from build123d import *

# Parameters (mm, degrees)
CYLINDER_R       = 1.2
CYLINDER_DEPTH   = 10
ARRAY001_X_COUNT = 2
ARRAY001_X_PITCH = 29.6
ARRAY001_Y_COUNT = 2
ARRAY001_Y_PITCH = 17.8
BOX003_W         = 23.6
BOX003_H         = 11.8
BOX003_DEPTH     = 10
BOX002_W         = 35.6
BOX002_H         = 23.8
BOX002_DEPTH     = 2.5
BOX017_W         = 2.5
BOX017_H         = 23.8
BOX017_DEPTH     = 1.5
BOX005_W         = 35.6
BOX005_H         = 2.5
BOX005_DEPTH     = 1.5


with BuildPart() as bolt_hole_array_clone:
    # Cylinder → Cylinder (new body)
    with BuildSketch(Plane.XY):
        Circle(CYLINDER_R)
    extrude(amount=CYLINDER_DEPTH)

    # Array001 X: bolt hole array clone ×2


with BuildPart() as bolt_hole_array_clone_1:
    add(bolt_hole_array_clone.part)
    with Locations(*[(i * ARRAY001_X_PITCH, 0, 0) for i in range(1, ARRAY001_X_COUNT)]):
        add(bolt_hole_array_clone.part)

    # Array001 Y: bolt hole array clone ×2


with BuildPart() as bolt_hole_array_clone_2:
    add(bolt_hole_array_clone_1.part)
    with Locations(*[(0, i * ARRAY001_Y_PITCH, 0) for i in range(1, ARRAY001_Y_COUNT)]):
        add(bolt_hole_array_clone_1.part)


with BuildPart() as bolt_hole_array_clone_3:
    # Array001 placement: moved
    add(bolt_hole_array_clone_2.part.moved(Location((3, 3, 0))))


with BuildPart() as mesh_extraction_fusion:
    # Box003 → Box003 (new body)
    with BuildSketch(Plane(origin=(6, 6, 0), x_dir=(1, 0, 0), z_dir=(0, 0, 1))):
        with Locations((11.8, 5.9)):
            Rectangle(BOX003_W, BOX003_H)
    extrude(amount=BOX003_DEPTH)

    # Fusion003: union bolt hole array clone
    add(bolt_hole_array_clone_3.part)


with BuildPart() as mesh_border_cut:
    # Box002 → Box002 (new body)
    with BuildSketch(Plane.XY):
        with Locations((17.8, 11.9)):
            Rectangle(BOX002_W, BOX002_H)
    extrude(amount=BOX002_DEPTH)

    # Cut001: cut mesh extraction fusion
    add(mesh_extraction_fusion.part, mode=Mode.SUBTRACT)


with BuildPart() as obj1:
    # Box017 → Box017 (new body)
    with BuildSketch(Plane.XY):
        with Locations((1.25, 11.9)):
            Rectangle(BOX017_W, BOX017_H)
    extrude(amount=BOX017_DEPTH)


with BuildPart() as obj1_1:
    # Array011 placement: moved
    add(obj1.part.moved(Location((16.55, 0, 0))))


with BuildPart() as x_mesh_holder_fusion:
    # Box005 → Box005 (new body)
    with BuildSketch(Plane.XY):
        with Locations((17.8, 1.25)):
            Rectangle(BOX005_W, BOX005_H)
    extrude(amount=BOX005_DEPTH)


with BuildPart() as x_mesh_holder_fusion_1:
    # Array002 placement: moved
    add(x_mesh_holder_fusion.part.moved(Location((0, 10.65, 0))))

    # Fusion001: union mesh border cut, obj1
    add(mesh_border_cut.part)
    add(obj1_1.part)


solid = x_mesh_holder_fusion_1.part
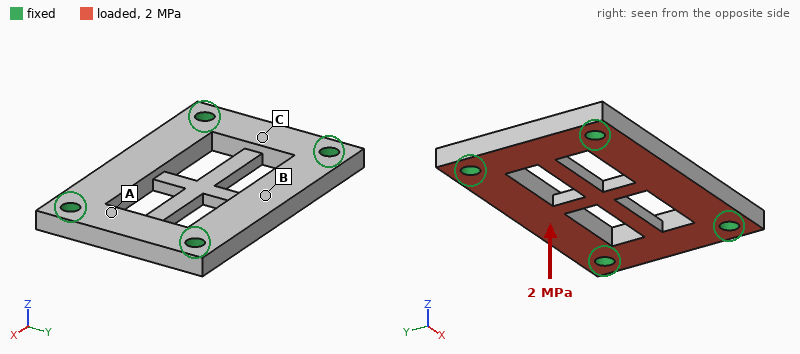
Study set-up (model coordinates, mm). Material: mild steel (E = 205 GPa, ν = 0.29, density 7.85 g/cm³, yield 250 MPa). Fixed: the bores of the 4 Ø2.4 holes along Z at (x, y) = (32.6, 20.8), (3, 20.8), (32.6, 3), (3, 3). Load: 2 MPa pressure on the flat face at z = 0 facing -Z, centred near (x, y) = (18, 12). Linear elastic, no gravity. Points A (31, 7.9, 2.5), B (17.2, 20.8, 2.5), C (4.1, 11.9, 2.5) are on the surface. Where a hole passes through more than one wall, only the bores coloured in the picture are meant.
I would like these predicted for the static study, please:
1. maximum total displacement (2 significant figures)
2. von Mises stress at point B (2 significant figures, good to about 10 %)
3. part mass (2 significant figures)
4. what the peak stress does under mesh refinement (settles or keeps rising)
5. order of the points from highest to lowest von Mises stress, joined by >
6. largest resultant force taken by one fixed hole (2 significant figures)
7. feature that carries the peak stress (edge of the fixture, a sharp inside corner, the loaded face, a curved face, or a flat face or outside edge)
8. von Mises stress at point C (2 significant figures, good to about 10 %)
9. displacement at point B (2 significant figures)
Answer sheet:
25 µm
83 MPa
12 g
keeps rising
B > C > A
320 N
edge of the fixture
47 MPa
16 µm
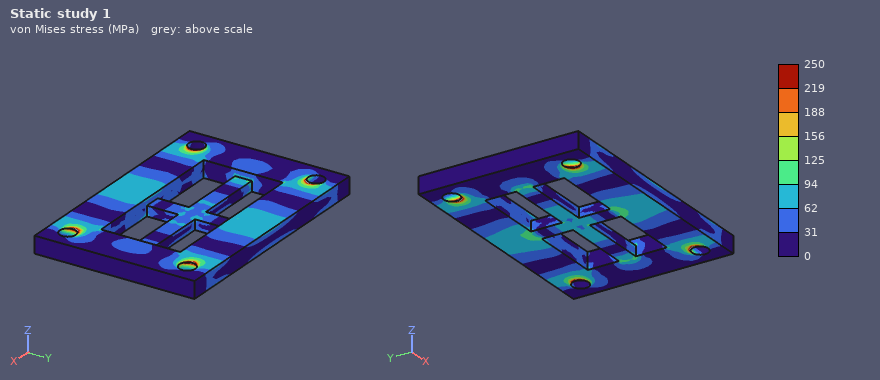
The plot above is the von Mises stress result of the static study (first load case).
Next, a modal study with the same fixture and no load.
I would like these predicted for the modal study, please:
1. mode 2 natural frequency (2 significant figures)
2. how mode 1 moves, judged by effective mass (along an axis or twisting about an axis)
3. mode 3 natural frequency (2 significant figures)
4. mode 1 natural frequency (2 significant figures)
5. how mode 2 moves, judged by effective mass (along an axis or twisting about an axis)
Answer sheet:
17 kHz
along Z
23 kHz
14 kHz
twisting about X
